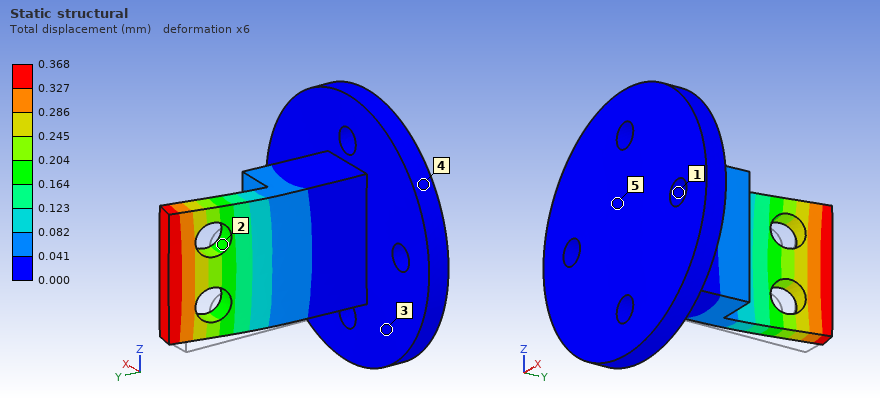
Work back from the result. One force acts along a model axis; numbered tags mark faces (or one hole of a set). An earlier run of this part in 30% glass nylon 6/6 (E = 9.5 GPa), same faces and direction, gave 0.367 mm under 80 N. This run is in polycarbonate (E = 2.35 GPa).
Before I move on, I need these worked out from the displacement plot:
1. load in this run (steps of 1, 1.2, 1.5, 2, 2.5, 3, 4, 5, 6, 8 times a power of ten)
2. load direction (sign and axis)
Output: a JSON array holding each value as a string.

["20 N", "+X"]
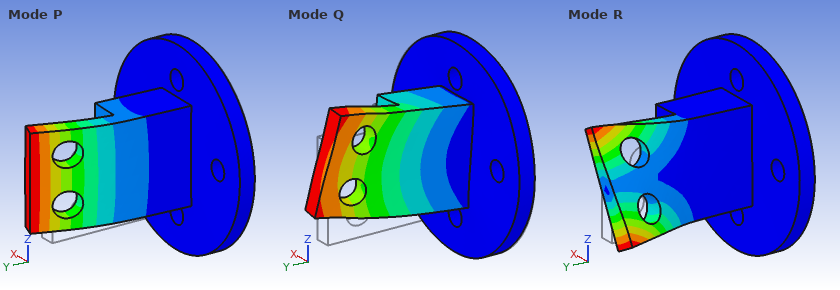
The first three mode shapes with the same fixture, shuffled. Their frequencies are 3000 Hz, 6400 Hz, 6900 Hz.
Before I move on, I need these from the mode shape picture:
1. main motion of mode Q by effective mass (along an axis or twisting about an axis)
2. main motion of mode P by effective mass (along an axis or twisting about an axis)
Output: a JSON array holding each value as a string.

["along Z", "along X"]
